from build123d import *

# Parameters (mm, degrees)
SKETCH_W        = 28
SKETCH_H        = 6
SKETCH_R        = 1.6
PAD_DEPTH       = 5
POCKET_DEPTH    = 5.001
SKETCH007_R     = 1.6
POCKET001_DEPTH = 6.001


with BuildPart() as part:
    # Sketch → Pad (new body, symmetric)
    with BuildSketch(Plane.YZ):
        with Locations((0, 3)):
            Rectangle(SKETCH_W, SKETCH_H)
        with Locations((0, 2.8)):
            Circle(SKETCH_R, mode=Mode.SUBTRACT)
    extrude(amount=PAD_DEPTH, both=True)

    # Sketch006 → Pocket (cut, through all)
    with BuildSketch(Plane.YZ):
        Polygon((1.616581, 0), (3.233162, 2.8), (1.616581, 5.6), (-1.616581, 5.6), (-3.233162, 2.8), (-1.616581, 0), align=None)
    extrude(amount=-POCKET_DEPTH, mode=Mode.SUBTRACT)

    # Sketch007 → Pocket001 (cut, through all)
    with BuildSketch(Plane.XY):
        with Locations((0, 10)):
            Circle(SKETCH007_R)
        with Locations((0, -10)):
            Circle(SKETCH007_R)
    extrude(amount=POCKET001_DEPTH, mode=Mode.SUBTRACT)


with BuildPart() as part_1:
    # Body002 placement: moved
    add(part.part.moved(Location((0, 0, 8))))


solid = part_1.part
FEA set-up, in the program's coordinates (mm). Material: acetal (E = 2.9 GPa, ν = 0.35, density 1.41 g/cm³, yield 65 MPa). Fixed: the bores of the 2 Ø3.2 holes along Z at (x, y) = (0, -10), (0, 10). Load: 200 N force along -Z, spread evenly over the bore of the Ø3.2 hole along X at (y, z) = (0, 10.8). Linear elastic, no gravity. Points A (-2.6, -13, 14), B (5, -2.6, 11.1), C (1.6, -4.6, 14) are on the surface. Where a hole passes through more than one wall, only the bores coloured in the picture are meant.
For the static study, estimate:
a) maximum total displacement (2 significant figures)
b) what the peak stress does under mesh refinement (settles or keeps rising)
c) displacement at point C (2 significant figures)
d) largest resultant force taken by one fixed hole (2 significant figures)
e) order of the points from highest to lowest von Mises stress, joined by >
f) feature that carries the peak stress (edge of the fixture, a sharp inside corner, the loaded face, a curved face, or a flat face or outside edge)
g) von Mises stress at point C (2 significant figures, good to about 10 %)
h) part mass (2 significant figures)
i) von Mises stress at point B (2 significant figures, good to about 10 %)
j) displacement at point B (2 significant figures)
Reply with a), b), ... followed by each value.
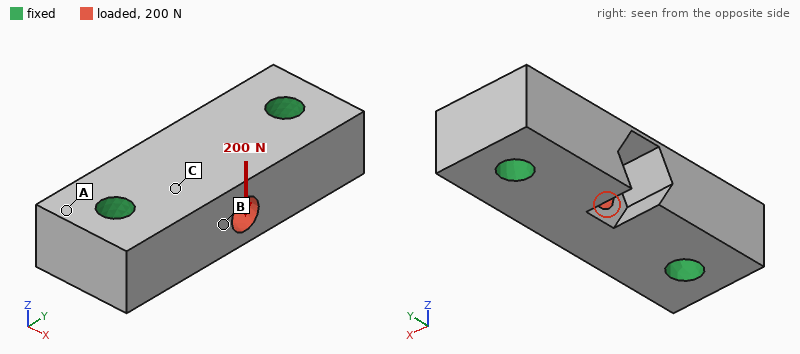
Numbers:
a) 59 µm
b) keeps rising
c) 25 µm
d) 100 N
e) B > C > A
f) edge of the fixture
g) 3.7 MPa
h) 2.0 g
i) 9.5 MPa
j) 45 µm
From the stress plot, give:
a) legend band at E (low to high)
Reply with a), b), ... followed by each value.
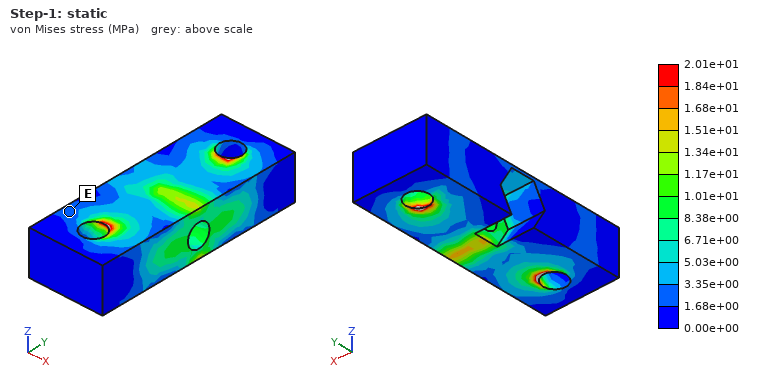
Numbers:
a) 1.68e+00 to 3.35e+00 MPa
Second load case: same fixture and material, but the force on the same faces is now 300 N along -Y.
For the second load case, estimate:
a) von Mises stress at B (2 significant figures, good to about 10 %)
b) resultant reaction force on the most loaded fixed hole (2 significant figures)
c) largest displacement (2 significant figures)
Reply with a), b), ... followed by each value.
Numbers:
a) 6.1 MPa
b) 150 N
c) 17 µm
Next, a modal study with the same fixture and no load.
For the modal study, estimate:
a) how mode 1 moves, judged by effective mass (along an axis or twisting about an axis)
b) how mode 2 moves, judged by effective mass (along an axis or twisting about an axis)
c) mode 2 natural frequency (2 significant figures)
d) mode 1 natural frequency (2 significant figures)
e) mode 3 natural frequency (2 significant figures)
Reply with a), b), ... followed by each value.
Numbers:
a) along X
b) along Z
c) 17 kHz
d) 16 kHz
e) 22 kHz
